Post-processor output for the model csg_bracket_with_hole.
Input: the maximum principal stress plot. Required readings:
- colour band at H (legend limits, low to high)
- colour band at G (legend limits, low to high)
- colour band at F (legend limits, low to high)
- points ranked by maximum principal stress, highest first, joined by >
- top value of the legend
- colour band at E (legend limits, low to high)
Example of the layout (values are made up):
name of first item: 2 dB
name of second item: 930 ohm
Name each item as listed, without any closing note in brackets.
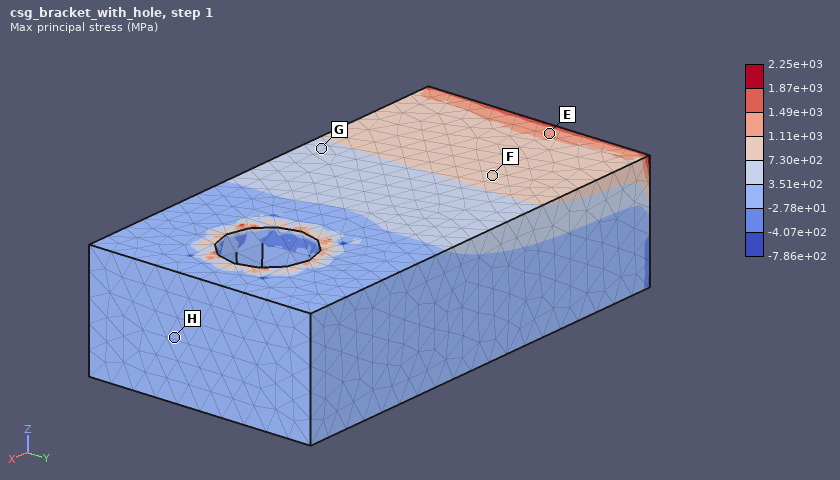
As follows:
colour band at H: -2.78e+01 to 3.51e+02 MPa
colour band at G: 3.51e+02 to 7.30e+02 MPa
colour band at F: 7.30e+02 to 1.11e+03 MPa
points ranked by maximum principal stress, highest first, joined by >: E > F > G > H
top value of the legend: 2.25e+03 MPa
colour band at E: 1.11e+03 to 1.49e+03 MPa
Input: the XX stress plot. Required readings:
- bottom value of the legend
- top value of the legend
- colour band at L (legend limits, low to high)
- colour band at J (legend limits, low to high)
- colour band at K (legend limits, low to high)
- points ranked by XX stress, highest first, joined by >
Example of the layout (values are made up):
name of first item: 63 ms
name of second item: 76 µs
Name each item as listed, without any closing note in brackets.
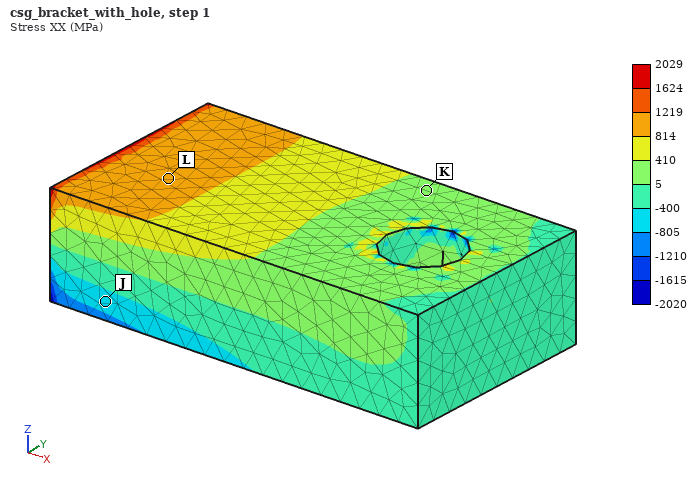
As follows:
bottom value of the legend: -2020 MPa
top value of the legend: 2029 MPa
colour band at L: 814 to 1219 MPa
colour band at J: -805 to -400 MPa
colour band at K: 5 to 410 MPa
points ranked by XX stress, highest first, joined by >: L > K > J
